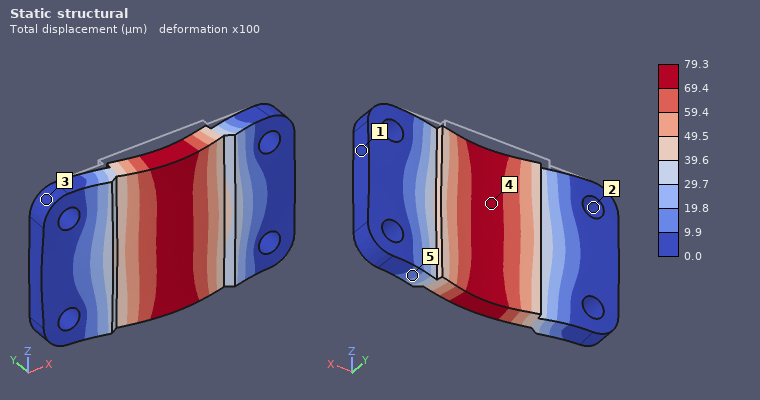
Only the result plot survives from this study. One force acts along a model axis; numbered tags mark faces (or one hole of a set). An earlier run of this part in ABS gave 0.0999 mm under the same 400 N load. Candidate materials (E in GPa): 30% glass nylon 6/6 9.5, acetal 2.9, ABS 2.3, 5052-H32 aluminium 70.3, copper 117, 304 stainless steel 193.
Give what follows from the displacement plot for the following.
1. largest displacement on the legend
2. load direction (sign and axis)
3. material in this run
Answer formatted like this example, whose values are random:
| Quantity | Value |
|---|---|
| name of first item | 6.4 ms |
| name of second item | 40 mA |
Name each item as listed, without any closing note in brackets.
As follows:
| Quantity | Value |
|---|---|
| largest displacement on the legend | 79.3 µm |
| load direction | -Y |
| material in this run | acetal |
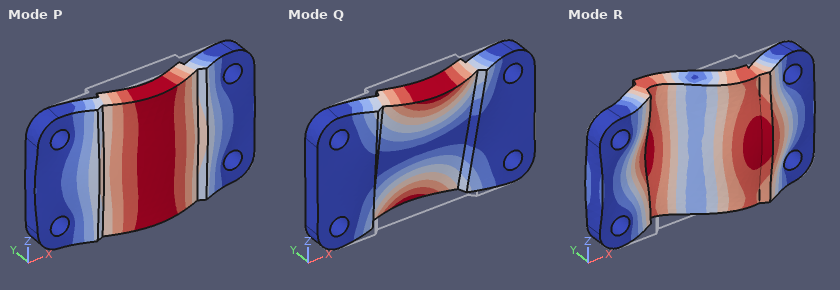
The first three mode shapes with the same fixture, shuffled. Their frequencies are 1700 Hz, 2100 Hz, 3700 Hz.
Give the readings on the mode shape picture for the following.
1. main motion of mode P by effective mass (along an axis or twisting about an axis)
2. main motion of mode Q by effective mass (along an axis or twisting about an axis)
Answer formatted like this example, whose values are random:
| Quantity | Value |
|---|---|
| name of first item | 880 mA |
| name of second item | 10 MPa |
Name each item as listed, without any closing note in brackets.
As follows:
| Quantity | Value |
|---|---|
| main motion of mode P by effective mass | along Y |
| main motion of mode Q by effective mass | twisting about X |
